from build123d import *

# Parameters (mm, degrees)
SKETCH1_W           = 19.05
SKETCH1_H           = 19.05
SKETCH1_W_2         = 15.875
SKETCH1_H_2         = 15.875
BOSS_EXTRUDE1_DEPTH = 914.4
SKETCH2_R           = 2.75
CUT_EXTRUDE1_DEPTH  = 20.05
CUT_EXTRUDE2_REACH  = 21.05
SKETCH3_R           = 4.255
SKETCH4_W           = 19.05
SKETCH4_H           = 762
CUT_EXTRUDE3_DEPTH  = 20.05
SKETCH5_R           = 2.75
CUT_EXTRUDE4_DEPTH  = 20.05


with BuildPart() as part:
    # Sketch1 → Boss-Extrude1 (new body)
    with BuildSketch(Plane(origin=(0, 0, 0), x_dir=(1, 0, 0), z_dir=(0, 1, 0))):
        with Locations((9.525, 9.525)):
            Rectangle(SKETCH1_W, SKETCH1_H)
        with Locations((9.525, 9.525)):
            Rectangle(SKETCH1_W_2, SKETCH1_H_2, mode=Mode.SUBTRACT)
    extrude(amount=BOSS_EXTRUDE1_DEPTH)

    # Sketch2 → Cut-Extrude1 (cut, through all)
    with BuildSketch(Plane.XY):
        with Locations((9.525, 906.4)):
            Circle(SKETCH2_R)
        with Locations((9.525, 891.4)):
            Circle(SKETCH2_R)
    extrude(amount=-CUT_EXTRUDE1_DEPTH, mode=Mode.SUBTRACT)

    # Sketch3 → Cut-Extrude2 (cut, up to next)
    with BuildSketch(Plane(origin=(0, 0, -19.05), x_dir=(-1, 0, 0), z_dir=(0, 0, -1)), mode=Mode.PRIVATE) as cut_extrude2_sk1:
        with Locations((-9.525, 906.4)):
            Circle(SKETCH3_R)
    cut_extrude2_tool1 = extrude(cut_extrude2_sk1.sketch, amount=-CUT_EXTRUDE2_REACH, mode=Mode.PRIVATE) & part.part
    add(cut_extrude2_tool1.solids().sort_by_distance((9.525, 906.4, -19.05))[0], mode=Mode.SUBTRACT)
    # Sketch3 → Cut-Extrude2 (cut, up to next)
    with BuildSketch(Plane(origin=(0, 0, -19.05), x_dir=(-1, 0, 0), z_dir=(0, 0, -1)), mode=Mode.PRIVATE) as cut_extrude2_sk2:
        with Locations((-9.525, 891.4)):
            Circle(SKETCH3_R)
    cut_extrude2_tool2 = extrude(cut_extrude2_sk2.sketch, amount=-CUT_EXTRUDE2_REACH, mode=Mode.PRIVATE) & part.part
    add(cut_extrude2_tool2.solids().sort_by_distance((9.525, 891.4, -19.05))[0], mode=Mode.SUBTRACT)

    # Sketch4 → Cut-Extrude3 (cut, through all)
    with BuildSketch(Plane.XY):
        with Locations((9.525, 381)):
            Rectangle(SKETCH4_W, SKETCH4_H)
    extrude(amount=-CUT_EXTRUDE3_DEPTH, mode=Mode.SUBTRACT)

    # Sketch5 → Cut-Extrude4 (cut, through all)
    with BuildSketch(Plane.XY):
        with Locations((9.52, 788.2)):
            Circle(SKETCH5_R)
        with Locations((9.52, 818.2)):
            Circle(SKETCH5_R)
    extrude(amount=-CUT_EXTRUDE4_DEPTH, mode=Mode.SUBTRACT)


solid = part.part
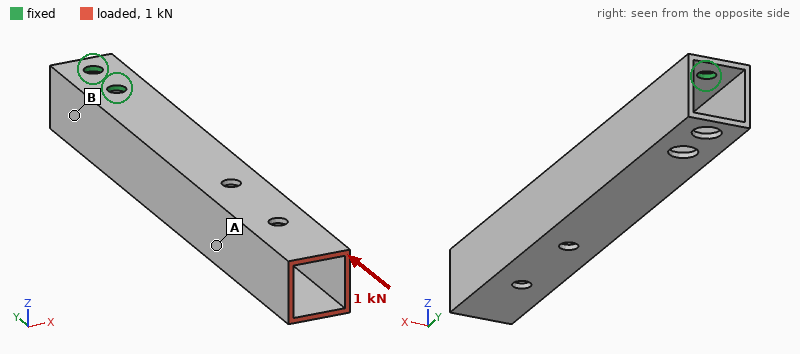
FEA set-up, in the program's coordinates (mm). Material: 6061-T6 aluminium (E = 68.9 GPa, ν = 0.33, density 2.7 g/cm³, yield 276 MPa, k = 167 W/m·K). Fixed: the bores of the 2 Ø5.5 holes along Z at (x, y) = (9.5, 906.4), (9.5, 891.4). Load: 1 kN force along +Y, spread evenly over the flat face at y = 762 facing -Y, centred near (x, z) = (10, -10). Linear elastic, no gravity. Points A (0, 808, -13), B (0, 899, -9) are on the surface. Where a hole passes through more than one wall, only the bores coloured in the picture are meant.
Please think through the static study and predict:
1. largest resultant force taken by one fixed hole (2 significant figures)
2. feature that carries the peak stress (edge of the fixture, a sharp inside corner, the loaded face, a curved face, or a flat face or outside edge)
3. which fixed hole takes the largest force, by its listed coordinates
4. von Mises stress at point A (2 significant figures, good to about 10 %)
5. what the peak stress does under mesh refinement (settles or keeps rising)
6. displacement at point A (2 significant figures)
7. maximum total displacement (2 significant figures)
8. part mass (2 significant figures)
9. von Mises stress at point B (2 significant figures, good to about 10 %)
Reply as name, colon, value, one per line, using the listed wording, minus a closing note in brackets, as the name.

largest resultant force taken by one fixed hole: 770 N
feature that carries the peak stress: edge of the fixture
which fixed hole takes the largest force, by its listed coordinates: (9.5, 891.4)
von Mises stress at point A: 9.8 MPa
what the peak stress does under mesh refinement: keeps rising
displacement at point A: 0.38 mm
maximum total displacement: 0.57 mm
part mass: 45 g
von Mises stress at point B: 23 MPa
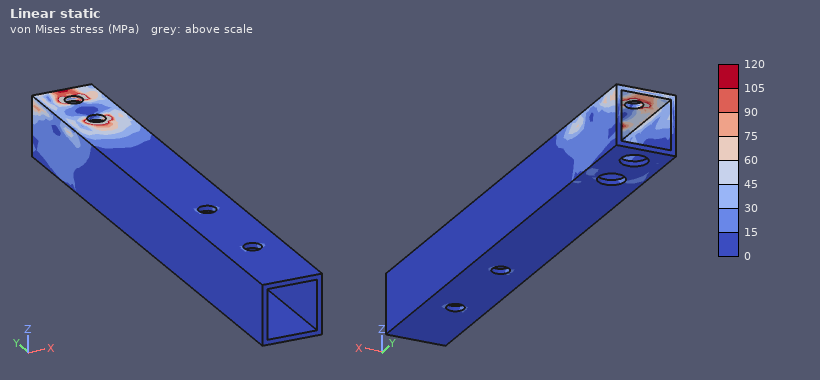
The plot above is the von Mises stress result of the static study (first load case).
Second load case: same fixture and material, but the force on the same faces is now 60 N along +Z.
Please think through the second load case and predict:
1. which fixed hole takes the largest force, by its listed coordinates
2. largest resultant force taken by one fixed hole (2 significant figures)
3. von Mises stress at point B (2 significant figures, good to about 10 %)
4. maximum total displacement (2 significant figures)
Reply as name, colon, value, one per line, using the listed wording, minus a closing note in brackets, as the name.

which fixed hole takes the largest force, by its listed coordinates: (9.5, 891.4)
largest resultant force taken by one fixed hole: 460 N
von Mises stress at point B: 20 MPa
maximum total displacement: 0.65 mm
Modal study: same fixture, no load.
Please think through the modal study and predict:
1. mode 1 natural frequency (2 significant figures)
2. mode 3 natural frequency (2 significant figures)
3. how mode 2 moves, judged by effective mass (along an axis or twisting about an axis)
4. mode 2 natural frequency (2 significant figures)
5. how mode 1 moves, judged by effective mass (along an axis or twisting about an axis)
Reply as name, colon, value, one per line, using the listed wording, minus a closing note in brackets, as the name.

mode 1 natural frequency: 430 Hz
mode 3 natural frequency: 1500 Hz
how mode 2 moves, judged by effective mass: along X
mode 2 natural frequency: 740 Hz
how mode 1 moves, judged by effective mass: along Z
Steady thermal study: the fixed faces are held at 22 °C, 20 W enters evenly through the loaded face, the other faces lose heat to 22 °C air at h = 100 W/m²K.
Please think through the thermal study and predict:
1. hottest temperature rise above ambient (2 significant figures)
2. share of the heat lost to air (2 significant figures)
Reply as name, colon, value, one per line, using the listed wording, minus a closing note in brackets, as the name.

hottest temperature rise above ambient: 40 K
share of the heat lost to air: 96 %
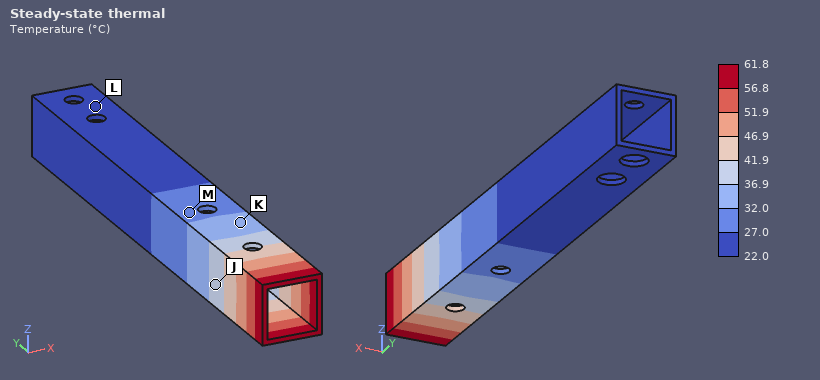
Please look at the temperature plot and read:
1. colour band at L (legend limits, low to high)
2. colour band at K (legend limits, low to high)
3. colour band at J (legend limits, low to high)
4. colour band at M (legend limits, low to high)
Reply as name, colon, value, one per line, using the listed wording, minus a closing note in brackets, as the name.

colour band at L: 22.0 to 27.0 °C
colour band at K: 32.0 to 36.9 °C
colour band at J: 36.9 to 41.9 °C
colour band at M: 27.0 to 32.0 °C
